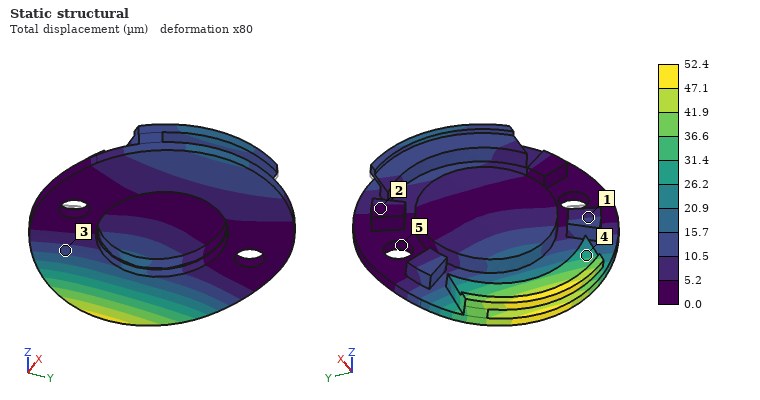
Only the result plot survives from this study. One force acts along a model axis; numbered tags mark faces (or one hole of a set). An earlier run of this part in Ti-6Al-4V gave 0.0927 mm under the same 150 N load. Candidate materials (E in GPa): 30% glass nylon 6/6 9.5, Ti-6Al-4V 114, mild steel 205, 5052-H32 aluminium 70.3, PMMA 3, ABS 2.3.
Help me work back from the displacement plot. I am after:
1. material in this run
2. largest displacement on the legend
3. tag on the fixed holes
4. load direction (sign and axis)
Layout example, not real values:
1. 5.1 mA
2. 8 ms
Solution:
1. mild steel
2. 52.4 µm
3. 5
4. -Z
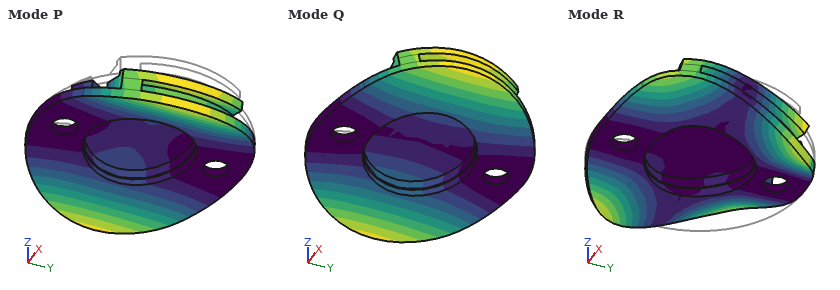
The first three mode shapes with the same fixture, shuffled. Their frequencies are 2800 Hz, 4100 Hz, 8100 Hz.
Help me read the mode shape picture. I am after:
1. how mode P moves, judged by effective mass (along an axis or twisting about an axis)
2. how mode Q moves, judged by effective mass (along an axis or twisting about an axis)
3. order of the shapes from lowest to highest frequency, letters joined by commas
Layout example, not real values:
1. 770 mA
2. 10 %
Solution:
1. along Z
2. twisting about Y
3. Q, P, R
